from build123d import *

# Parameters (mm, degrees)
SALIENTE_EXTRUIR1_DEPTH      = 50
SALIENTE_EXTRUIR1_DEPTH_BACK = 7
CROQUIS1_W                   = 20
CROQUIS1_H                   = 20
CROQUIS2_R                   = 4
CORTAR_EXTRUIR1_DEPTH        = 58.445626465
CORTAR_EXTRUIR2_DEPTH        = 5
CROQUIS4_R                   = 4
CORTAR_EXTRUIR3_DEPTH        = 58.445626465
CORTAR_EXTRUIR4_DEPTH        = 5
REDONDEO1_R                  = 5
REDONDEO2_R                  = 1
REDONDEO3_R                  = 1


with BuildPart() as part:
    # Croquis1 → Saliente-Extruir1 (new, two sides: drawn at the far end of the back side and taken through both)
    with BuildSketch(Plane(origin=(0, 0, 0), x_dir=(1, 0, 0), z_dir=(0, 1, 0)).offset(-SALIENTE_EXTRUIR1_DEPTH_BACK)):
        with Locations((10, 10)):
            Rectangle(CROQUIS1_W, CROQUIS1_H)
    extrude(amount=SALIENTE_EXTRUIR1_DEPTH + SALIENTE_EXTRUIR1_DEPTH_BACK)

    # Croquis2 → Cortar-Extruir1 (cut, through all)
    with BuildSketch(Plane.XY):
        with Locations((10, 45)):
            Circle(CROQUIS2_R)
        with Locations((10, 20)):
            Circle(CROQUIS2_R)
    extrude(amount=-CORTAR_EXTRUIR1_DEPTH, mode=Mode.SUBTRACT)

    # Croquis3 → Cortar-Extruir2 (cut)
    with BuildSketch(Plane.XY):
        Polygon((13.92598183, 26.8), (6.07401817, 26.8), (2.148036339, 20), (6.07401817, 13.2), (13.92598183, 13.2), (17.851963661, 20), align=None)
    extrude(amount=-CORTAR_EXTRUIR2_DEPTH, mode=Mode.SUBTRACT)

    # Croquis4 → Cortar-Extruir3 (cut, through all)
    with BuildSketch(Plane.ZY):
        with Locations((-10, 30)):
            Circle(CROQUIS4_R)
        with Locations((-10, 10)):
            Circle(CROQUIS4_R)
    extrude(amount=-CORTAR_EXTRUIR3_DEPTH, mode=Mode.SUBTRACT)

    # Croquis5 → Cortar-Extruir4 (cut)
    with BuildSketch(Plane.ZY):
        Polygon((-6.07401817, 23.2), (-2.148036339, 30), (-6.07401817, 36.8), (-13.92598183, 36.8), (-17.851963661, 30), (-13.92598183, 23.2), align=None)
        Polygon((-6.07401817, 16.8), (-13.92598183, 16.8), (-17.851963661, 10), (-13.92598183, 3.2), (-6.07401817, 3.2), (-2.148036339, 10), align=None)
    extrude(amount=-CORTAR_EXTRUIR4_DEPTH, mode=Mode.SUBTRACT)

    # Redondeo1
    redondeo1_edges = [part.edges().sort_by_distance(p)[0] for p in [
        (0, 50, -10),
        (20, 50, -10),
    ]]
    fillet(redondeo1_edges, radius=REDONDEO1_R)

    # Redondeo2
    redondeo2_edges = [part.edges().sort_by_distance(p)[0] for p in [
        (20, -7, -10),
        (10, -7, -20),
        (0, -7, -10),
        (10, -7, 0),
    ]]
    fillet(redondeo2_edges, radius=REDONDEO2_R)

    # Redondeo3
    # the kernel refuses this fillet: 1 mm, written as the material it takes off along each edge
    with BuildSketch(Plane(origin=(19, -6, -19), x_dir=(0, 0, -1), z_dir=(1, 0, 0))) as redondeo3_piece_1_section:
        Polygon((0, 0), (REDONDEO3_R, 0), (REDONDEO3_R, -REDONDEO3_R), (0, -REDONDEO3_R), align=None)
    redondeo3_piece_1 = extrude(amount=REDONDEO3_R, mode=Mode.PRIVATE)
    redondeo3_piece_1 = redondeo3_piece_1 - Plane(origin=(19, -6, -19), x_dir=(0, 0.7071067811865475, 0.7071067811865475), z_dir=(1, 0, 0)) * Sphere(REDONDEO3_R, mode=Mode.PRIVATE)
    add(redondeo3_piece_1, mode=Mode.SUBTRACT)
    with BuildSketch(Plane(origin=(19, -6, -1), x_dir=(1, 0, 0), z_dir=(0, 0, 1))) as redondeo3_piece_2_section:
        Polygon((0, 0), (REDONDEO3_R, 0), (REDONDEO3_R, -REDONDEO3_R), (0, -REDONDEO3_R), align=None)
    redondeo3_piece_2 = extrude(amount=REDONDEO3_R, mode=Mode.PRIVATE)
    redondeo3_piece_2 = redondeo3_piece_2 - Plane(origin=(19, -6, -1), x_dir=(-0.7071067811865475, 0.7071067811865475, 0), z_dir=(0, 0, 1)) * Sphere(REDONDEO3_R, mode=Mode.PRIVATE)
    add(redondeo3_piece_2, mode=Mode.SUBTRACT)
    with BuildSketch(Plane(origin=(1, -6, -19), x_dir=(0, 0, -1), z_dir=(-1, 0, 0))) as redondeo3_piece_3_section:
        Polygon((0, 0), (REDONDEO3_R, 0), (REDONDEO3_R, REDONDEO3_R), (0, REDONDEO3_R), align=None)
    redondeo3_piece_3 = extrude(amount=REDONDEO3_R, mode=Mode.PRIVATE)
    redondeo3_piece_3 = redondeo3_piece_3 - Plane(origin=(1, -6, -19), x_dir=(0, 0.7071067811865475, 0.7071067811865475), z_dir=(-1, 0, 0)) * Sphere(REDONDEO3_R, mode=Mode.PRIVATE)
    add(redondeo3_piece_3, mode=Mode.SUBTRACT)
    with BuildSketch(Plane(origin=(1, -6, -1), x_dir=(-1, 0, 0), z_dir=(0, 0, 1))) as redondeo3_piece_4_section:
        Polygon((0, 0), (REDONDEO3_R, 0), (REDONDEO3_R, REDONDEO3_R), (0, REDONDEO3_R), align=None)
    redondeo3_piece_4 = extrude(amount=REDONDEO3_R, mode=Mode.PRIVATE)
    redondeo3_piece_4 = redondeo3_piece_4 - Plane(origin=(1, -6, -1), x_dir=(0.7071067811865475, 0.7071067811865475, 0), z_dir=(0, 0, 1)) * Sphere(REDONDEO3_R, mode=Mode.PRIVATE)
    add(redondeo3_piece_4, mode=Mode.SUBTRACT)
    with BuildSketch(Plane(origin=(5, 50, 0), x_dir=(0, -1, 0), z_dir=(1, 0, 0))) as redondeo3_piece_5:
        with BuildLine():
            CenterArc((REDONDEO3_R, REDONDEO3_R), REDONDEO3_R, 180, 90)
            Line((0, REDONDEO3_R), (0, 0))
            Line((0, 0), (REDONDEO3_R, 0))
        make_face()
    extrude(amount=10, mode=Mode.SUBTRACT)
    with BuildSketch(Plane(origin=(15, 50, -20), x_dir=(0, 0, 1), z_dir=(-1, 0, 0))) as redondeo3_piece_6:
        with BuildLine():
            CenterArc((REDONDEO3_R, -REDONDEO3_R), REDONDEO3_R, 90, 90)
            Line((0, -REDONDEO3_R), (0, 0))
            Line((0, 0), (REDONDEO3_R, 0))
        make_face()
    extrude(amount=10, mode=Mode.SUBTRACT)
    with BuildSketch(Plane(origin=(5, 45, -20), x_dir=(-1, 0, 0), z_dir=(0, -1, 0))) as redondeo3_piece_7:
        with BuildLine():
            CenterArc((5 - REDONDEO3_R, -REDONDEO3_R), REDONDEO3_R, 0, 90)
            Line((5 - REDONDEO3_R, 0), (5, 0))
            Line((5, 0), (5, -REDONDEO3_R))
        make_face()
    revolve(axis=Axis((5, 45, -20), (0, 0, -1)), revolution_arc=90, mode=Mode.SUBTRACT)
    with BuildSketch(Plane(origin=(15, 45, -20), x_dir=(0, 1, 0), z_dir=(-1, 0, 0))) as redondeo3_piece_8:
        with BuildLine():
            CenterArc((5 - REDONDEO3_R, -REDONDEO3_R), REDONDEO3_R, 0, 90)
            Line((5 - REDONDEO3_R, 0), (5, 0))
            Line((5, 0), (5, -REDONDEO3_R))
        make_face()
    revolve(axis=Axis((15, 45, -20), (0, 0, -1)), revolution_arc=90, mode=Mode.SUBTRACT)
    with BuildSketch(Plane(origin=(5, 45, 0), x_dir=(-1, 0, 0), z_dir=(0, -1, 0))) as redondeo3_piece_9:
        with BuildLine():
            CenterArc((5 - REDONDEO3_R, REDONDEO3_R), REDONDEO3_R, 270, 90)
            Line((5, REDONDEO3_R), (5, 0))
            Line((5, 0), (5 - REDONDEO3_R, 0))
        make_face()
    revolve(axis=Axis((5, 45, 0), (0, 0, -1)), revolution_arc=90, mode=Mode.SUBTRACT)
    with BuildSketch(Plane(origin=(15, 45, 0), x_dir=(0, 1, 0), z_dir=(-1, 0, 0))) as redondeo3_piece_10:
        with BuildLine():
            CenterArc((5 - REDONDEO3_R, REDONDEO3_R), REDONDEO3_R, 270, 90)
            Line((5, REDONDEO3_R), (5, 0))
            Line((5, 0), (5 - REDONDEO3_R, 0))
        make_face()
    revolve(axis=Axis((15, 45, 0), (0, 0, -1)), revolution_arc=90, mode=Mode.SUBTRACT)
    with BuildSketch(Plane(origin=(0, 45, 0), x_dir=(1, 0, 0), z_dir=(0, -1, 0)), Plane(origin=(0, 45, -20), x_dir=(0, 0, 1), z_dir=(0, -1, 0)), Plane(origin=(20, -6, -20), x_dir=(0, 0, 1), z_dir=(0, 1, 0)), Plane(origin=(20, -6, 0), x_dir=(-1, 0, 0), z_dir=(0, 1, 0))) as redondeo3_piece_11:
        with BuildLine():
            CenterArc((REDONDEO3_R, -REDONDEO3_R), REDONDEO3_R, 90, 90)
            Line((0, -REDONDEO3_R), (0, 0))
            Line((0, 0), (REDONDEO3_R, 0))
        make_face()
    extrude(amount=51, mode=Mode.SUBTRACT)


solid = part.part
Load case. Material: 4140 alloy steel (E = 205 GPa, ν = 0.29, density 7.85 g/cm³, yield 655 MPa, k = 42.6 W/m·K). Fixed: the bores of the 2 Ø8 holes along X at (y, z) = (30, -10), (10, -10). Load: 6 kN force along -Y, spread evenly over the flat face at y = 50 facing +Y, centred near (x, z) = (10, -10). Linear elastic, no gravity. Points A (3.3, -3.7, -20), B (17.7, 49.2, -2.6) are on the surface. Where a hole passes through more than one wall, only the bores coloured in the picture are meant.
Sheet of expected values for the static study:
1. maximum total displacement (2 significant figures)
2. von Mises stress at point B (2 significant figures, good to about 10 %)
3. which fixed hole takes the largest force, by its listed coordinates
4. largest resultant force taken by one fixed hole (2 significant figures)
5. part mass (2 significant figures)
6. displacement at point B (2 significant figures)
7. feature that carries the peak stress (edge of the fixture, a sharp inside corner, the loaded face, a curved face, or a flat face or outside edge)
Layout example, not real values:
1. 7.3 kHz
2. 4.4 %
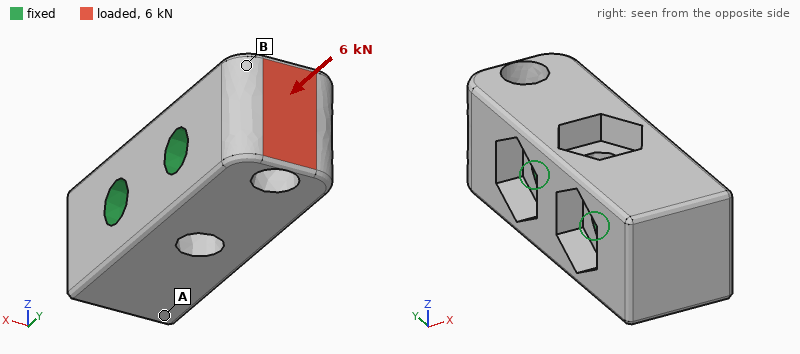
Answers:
1. 11 µm
2. 34 MPa
3. (30, -10)
4. 5.5 kN
5. 130 g
6. 1.7 µm
7. the loaded face
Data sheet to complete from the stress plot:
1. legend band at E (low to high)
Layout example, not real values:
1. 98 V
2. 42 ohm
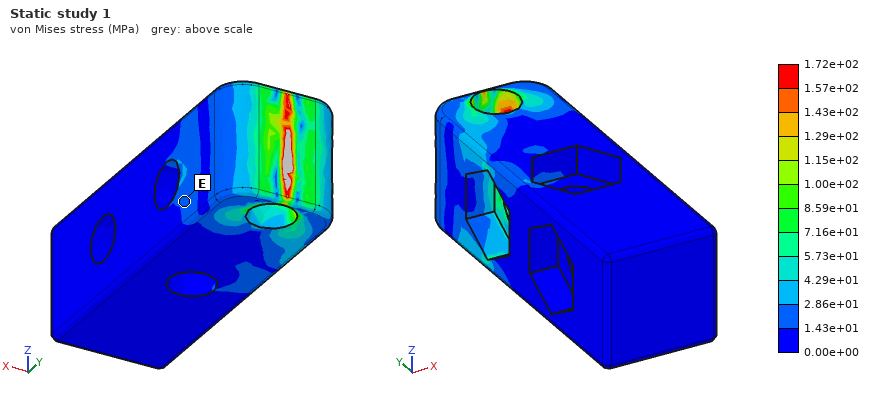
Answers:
1. 1.43e+01 to 2.86e+01 MPa
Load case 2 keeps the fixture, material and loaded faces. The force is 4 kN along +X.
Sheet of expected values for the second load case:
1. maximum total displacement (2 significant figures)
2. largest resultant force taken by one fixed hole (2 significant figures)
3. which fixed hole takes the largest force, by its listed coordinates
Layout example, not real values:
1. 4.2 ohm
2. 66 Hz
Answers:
1. 16 µm
2. 4.4 kN
3. (30, -10)
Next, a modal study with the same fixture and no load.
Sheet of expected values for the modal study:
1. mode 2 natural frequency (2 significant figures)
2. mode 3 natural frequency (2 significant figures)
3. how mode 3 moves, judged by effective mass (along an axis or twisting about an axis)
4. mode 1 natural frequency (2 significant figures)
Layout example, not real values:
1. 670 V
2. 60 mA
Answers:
1. 25 kHz
2. 27 kHz
3. along Z
4. 24 kHz
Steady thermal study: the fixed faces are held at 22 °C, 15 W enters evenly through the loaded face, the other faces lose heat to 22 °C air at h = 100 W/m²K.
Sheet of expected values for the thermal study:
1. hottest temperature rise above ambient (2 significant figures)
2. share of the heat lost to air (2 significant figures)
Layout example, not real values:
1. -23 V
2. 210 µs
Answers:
1. 33 K
2. 16 %
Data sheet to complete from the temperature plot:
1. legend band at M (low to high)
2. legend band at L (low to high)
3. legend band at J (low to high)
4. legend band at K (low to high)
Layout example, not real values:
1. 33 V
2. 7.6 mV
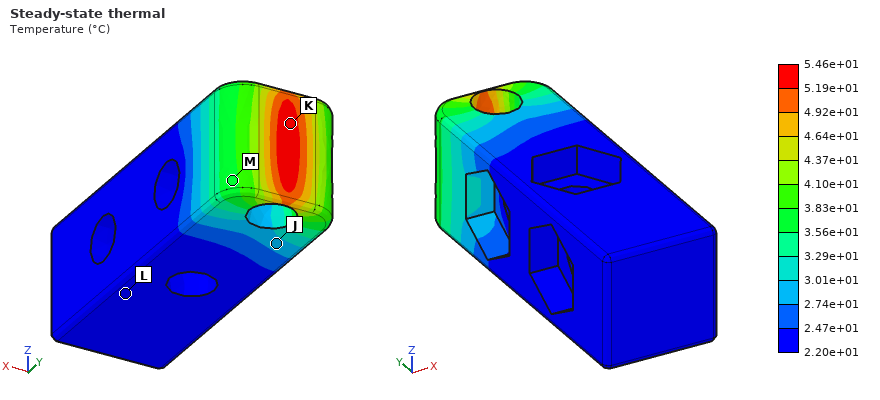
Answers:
1. 3.56e+01 to 3.83e+01 °C
2. 2.20e+01 to 2.47e+01 °C
3. 2.74e+01 to 3.01e+01 °C
4. 5.19e+01 to 5.46e+01 °C
